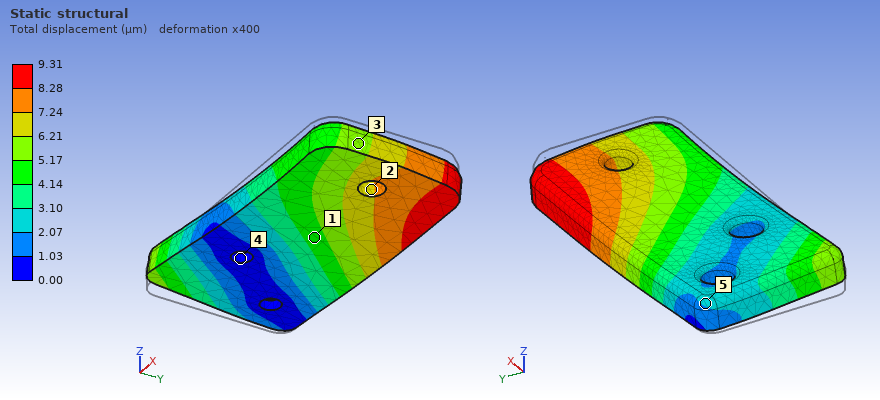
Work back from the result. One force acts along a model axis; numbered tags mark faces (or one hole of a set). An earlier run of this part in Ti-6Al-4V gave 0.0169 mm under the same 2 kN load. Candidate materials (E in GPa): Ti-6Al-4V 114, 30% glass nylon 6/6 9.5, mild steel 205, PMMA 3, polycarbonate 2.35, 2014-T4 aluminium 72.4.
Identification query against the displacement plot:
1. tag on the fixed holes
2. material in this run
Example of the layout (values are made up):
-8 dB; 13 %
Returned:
4; mild steel
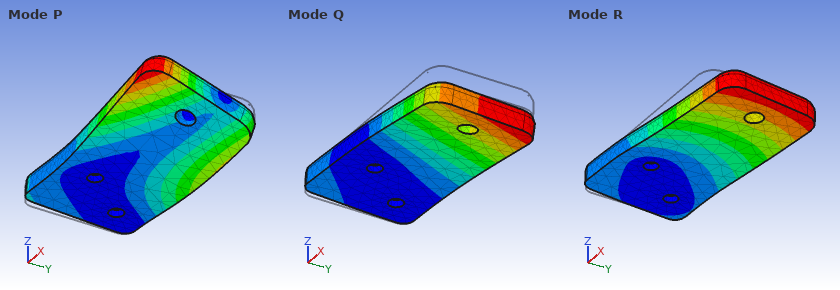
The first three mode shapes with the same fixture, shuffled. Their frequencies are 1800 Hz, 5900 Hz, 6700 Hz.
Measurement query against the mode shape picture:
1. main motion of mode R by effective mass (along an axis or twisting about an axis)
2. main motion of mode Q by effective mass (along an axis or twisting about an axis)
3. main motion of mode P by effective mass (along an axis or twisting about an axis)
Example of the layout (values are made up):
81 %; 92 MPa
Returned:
along Y; along Z; twisting about X
